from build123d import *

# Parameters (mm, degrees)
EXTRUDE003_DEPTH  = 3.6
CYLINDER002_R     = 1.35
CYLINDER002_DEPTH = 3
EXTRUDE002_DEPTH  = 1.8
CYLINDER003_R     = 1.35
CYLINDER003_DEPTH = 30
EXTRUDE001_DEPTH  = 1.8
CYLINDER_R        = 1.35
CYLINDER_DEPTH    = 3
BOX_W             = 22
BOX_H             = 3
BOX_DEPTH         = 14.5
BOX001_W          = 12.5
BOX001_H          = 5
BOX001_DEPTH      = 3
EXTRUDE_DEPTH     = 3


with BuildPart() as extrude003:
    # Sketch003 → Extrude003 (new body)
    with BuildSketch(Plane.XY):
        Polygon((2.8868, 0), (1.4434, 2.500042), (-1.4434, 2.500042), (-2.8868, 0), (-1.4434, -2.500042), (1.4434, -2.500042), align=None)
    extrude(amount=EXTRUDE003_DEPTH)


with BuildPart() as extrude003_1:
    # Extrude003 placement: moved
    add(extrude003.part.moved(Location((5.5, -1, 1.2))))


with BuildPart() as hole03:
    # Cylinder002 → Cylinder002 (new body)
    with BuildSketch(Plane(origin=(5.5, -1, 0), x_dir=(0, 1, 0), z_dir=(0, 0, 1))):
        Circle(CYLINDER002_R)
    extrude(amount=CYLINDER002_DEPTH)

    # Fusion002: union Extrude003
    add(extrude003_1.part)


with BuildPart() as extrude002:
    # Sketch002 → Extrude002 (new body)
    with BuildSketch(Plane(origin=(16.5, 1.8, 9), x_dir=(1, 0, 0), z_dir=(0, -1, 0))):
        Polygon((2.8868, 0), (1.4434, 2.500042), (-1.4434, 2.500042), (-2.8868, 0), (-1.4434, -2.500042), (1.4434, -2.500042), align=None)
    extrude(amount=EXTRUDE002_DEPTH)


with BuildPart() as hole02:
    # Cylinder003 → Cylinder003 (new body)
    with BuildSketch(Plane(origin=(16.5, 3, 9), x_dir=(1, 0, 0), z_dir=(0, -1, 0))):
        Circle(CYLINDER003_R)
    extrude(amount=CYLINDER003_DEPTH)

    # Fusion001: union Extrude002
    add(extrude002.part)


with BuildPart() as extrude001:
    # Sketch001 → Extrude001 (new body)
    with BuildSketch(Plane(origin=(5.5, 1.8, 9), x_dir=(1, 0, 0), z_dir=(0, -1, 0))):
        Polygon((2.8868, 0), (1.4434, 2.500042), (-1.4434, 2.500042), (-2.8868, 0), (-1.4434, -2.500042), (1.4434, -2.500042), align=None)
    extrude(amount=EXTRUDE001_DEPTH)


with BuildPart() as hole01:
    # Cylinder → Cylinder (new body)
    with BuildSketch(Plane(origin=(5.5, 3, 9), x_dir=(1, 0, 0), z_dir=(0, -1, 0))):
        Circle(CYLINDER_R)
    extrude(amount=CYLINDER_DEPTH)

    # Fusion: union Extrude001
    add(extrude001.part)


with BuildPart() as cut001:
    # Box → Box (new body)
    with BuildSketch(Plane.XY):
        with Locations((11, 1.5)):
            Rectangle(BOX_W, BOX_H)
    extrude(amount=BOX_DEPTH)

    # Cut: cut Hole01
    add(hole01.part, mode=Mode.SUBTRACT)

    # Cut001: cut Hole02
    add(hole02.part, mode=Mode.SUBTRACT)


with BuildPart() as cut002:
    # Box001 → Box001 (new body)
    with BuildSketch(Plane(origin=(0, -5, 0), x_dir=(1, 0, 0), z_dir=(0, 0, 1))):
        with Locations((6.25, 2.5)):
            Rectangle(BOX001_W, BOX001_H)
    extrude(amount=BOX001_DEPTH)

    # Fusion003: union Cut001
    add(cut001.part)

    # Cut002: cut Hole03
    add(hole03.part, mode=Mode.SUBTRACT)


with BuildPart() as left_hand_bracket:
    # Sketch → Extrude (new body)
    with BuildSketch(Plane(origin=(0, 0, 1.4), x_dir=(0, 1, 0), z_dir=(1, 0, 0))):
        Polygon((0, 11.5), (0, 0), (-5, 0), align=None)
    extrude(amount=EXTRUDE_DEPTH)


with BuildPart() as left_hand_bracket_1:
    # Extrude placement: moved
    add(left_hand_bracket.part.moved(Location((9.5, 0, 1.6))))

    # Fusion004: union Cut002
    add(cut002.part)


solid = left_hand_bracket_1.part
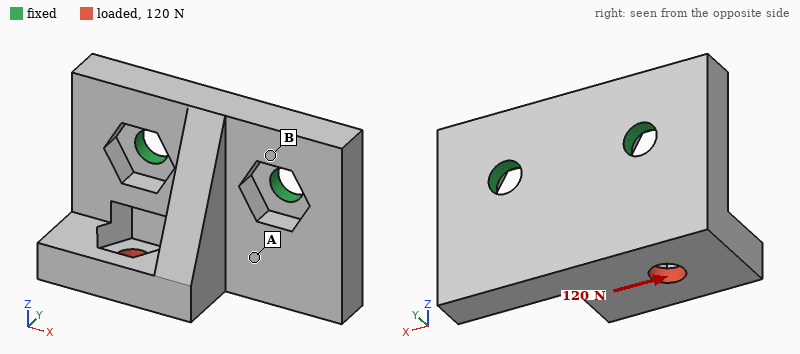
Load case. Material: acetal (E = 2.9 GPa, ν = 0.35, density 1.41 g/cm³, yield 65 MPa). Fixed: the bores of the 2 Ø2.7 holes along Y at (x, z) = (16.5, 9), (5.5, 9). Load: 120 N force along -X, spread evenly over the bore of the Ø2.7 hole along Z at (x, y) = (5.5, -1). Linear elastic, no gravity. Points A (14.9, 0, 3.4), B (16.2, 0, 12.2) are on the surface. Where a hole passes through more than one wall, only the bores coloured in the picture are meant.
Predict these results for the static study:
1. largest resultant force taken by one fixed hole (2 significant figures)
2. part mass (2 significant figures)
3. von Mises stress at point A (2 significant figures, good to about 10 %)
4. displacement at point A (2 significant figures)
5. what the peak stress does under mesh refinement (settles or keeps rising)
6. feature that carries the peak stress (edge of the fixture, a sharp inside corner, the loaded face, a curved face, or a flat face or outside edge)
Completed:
110 N
1.5 g
7.0 MPa
0.030 mm
keeps rising
edge of the fixture
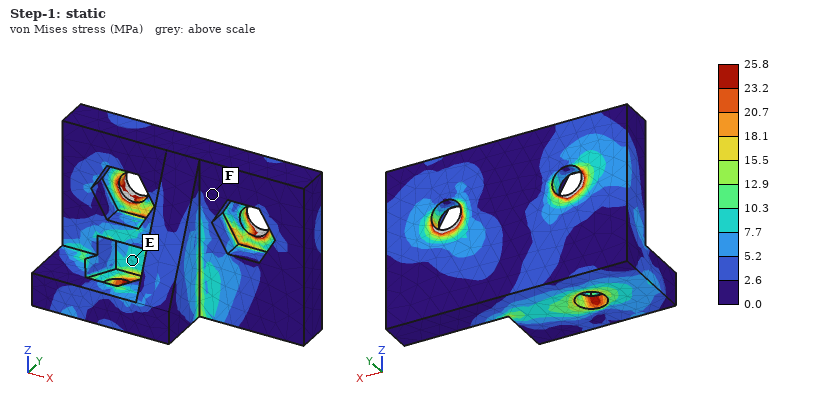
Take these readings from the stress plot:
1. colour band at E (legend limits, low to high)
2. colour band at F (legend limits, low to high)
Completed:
7.7 to 10.3 MPa
0.0 to 2.6 MPa
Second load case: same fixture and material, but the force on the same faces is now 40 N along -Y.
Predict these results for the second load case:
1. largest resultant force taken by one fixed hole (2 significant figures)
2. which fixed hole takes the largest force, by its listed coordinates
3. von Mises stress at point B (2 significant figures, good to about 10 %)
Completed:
39 N
(5.5, 9)
4.7 MPa
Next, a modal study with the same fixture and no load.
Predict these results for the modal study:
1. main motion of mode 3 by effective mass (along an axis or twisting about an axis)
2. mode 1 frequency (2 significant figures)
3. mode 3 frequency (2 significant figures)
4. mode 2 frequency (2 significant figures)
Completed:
along X
3100 Hz
9400 Hz
6200 Hz
